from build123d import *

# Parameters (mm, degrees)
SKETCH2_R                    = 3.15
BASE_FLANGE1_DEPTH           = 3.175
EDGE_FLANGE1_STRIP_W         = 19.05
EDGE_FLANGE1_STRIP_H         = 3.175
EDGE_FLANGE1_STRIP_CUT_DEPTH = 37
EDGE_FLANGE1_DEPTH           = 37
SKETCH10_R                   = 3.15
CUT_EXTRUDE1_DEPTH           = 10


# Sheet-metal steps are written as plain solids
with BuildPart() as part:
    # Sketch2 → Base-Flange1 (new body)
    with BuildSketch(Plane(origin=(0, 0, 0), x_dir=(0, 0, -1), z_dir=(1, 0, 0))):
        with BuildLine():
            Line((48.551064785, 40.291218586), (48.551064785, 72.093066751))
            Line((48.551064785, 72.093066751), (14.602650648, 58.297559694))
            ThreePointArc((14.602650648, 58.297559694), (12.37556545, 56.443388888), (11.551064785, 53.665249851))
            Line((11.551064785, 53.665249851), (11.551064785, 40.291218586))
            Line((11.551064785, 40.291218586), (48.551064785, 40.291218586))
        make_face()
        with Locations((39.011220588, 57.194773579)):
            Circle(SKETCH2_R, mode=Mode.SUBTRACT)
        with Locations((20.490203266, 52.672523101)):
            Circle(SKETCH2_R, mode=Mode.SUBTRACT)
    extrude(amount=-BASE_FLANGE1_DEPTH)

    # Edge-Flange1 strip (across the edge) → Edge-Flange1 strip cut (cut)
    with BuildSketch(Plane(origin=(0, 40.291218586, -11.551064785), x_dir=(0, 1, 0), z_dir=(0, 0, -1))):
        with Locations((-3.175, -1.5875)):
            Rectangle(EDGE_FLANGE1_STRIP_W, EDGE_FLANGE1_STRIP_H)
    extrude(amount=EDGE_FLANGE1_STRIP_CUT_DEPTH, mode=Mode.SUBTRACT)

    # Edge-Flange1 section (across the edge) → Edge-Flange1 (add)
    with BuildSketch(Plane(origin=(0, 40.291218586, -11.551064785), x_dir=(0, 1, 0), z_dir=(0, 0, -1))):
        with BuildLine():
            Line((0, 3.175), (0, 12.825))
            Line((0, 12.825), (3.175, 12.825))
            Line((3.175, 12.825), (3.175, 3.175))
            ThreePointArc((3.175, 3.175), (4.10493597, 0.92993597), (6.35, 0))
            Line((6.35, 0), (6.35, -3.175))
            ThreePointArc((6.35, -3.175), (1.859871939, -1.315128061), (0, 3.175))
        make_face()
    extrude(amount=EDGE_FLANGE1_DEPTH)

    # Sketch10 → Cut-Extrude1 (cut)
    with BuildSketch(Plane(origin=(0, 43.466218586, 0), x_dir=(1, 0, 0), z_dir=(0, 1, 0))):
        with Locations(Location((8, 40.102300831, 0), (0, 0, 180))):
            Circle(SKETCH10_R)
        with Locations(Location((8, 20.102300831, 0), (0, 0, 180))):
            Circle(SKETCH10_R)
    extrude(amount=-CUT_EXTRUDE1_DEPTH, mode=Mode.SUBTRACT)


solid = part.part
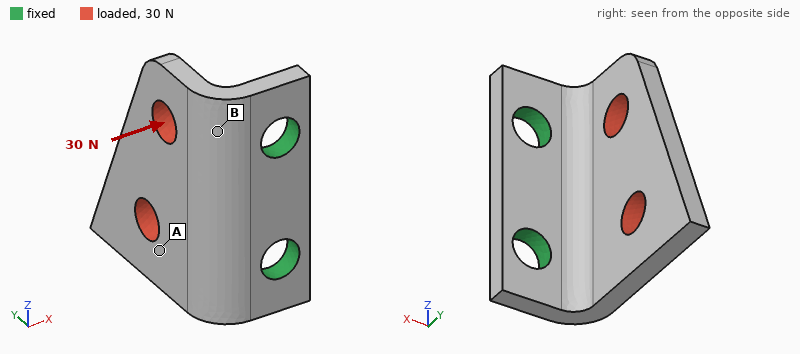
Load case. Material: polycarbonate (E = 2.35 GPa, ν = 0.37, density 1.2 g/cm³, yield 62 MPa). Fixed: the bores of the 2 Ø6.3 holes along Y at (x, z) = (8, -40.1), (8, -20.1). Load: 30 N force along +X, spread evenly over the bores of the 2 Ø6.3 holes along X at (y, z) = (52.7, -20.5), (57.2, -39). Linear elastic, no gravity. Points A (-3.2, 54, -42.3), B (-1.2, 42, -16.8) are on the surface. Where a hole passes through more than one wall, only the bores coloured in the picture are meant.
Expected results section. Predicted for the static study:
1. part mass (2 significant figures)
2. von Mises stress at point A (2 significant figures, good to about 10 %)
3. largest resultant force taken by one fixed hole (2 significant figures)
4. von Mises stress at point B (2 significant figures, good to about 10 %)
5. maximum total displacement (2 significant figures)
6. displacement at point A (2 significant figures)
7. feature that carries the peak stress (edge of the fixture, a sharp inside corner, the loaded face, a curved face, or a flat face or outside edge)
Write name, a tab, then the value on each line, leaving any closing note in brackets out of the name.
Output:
part mass	4.5 g
von Mises stress at point A	1.6 MPa
largest resultant force taken by one fixed hole	16 N
von Mises stress at point B	3.6 MPa
maximum total displacement	0.58 mm
displacement at point A	0.21 mm
feature that carries the peak stress	a flat face or outside edge
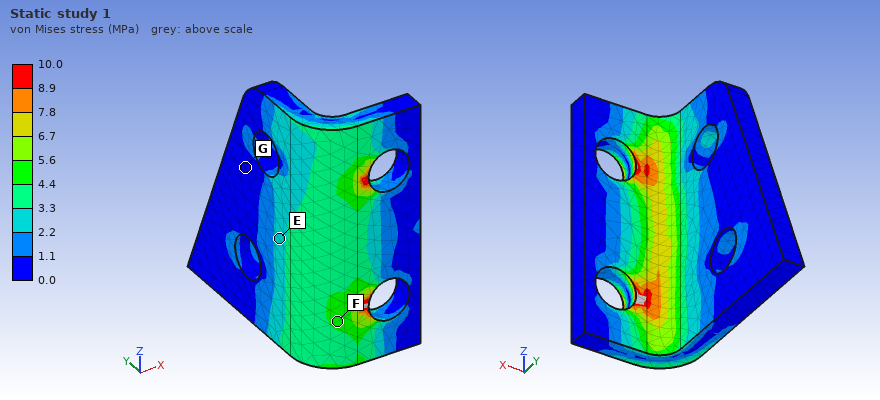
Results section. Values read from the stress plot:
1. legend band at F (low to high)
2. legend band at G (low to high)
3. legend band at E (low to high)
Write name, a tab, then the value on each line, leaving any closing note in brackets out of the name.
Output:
legend band at F	4.4 to 5.6 MPa
legend band at G	0.0 to 1.1 MPa
legend band at E	2.2 to 3.3 MPa
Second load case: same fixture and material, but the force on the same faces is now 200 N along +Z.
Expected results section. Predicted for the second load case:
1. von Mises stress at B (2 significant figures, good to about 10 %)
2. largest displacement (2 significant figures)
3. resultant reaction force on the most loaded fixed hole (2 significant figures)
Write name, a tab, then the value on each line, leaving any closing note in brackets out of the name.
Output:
von Mises stress at B	3.2 MPa
largest displacement	0.51 mm
resultant reaction force on the most loaded fixed hole	160 N
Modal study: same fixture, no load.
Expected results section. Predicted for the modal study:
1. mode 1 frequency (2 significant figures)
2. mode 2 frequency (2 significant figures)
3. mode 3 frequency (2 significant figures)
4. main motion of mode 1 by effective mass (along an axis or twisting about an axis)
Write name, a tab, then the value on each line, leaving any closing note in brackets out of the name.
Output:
mode 1 frequency	890 Hz
mode 2 frequency	2000 Hz
mode 3 frequency	2900 Hz
main motion of mode 1 by effective mass	along X
